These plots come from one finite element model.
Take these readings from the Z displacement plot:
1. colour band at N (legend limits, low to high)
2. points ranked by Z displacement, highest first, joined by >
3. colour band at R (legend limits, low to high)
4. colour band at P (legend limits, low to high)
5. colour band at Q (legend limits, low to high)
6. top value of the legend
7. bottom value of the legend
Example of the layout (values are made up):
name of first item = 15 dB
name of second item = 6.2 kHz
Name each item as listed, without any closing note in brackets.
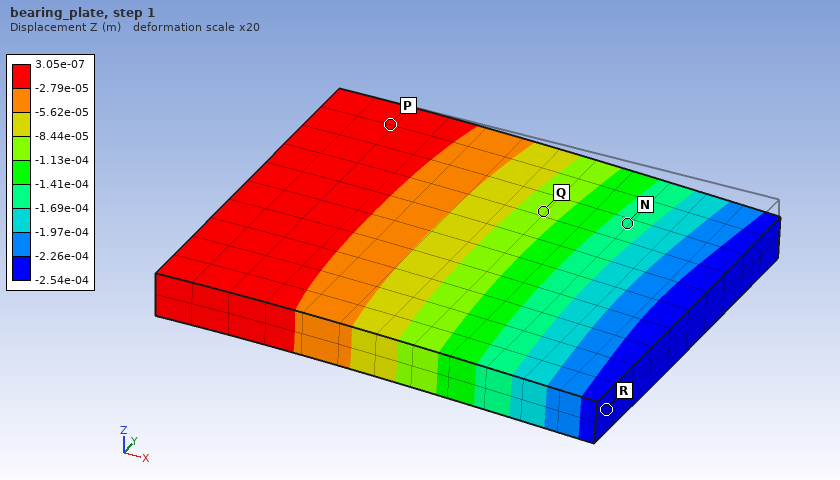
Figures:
colour band at N = -1.69e-04 to -1.41e-04 m
points ranked by Z displacement, highest first, joined by > = P > Q > N > R
colour band at R = -2.54e-04 to -2.26e-04 m
colour band at P = -2.79e-05 to 3.05e-07 m
colour band at Q = -1.13e-04 to -8.44e-05 m
top value of the legend = 3.05e-07 m
bottom value of the legend = -2.54e-04 m
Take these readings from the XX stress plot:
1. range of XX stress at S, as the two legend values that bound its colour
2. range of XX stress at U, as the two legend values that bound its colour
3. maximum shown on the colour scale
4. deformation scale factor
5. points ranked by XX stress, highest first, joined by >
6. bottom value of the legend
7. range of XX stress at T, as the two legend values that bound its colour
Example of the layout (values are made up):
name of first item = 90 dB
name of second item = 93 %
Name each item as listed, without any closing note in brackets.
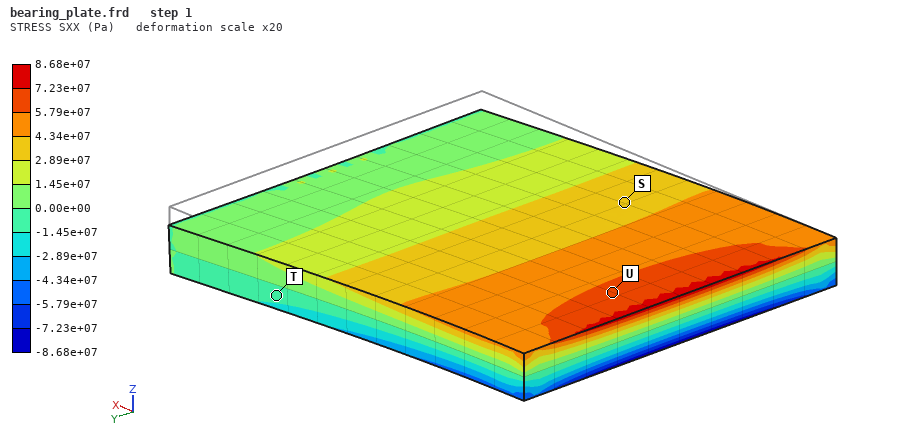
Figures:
range of XX stress at S, as the two legend values that bound its colour = 2.89e+07 to 4.34e+07 Pa
range of XX stress at U, as the two legend values that bound its colour = 5.79e+07 to 7.23e+07 Pa
maximum shown on the colour scale = 8.68e+07 Pa
deformation scale factor = 20
points ranked by XX stress, highest first, joined by > = U > S > T
bottom value of the legend = -8.68e+07 Pa
range of XX stress at T, as the two legend values that bound its colour = -1.45e+07 to 0.00e+00 Pa
